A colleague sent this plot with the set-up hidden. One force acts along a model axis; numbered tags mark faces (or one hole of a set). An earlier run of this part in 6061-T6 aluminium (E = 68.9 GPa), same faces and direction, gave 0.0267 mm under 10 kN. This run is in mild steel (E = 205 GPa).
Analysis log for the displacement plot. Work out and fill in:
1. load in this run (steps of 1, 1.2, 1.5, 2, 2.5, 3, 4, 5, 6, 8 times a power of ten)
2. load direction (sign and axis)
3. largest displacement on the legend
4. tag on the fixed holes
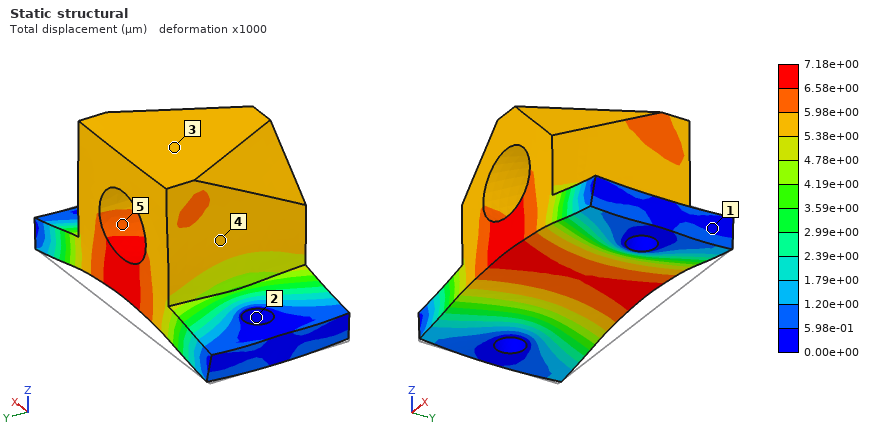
8 kN
+Z
7.18e+00 µm
2
